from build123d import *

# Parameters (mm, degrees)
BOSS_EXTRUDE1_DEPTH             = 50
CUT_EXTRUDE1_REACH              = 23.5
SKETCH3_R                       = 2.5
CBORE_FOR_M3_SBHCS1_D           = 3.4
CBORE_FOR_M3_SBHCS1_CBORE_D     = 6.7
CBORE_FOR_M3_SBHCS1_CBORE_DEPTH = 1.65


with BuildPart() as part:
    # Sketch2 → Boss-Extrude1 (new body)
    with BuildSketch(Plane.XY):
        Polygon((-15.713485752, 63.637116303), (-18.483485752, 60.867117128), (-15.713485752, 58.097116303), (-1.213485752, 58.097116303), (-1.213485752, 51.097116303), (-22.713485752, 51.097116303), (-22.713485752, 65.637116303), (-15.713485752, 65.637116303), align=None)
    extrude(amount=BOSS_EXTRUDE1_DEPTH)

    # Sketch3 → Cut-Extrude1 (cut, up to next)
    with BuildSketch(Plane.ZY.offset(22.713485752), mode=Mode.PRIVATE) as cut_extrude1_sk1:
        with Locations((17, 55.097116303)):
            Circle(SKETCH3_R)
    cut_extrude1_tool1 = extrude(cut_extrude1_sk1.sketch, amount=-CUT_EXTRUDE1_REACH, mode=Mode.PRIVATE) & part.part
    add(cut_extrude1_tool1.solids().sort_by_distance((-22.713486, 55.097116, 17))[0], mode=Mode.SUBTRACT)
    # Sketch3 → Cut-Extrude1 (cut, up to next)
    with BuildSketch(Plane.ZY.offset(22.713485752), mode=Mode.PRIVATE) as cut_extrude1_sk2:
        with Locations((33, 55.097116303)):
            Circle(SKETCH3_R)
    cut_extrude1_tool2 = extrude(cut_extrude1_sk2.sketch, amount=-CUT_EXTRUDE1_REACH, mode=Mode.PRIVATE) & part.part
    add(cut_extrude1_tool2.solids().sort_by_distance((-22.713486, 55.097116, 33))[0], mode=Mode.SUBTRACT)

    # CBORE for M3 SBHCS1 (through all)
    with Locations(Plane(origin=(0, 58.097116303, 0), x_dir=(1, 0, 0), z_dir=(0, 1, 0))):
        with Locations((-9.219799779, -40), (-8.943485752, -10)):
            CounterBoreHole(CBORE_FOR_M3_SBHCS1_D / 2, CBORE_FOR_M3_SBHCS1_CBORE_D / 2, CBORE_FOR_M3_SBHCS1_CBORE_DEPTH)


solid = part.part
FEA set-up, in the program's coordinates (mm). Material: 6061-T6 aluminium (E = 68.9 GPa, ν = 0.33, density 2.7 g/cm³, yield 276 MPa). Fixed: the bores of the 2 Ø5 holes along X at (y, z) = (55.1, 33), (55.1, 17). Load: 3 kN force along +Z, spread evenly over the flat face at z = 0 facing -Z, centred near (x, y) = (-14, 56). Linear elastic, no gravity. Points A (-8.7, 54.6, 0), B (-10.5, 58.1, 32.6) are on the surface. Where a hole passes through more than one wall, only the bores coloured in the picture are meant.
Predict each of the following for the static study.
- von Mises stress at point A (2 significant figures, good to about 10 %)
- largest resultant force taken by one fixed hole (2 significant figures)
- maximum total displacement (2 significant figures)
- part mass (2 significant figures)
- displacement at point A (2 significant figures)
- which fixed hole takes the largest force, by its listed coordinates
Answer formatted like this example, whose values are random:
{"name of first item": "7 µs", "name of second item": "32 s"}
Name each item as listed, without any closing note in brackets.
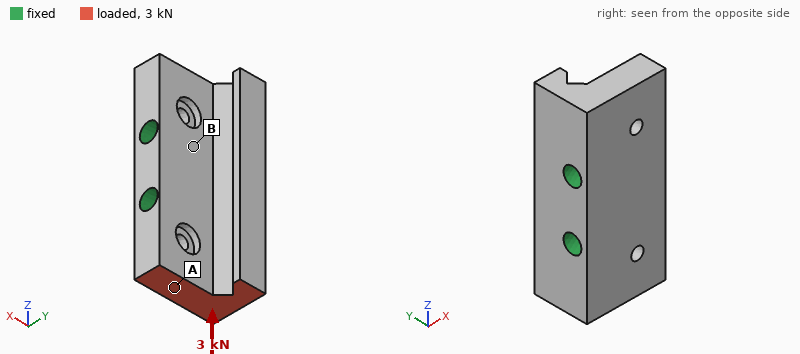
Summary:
{"von Mises stress at point A": "14 MPa", "largest resultant force taken by one fixed hole": "2.8 kN", "maximum total displacement": "6.8 µm", "part mass": "24 g", "displacement at point A": "4.4 µm", "which fixed hole takes the largest force, by its listed coordinates": "(55.1, 17)"}
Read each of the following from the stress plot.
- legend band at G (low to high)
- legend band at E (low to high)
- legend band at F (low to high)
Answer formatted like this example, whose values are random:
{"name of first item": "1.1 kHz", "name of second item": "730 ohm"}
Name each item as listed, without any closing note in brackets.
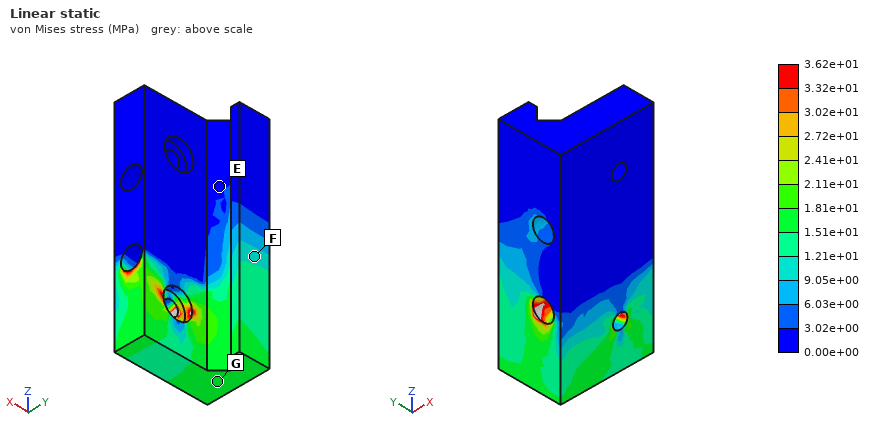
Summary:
{"legend band at G": "1.51e+01 to 1.81e+01 MPa", "legend band at E": "0.00e+00 to 3.02e+00 MPa", "legend band at F": "9.05e+00 to 1.21e+01 MPa"}
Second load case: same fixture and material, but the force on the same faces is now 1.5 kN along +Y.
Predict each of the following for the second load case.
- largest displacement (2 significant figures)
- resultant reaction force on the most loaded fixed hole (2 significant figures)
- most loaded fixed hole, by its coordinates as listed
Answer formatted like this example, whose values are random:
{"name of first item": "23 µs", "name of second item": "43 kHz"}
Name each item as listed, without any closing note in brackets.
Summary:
{"largest displacement": "41 µm", "resultant reaction force on the most loaded fixed hole": "2.0 kN", "most loaded fixed hole, by its coordinates as listed": "(55.1, 17)"}
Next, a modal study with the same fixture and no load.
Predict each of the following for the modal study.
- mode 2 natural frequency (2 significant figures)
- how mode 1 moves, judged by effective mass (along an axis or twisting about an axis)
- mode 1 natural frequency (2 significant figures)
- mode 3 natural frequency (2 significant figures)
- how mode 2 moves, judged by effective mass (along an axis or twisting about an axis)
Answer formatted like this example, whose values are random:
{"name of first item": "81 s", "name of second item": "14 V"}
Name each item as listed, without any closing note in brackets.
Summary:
{"mode 2 natural frequency": "22 kHz", "how mode 1 moves, judged by effective mass": "twisting about X", "mode 1 natural frequency": "21 kHz", "mode 3 natural frequency": "26 kHz", "how mode 2 moves, judged by effective mass": "along Y"}
